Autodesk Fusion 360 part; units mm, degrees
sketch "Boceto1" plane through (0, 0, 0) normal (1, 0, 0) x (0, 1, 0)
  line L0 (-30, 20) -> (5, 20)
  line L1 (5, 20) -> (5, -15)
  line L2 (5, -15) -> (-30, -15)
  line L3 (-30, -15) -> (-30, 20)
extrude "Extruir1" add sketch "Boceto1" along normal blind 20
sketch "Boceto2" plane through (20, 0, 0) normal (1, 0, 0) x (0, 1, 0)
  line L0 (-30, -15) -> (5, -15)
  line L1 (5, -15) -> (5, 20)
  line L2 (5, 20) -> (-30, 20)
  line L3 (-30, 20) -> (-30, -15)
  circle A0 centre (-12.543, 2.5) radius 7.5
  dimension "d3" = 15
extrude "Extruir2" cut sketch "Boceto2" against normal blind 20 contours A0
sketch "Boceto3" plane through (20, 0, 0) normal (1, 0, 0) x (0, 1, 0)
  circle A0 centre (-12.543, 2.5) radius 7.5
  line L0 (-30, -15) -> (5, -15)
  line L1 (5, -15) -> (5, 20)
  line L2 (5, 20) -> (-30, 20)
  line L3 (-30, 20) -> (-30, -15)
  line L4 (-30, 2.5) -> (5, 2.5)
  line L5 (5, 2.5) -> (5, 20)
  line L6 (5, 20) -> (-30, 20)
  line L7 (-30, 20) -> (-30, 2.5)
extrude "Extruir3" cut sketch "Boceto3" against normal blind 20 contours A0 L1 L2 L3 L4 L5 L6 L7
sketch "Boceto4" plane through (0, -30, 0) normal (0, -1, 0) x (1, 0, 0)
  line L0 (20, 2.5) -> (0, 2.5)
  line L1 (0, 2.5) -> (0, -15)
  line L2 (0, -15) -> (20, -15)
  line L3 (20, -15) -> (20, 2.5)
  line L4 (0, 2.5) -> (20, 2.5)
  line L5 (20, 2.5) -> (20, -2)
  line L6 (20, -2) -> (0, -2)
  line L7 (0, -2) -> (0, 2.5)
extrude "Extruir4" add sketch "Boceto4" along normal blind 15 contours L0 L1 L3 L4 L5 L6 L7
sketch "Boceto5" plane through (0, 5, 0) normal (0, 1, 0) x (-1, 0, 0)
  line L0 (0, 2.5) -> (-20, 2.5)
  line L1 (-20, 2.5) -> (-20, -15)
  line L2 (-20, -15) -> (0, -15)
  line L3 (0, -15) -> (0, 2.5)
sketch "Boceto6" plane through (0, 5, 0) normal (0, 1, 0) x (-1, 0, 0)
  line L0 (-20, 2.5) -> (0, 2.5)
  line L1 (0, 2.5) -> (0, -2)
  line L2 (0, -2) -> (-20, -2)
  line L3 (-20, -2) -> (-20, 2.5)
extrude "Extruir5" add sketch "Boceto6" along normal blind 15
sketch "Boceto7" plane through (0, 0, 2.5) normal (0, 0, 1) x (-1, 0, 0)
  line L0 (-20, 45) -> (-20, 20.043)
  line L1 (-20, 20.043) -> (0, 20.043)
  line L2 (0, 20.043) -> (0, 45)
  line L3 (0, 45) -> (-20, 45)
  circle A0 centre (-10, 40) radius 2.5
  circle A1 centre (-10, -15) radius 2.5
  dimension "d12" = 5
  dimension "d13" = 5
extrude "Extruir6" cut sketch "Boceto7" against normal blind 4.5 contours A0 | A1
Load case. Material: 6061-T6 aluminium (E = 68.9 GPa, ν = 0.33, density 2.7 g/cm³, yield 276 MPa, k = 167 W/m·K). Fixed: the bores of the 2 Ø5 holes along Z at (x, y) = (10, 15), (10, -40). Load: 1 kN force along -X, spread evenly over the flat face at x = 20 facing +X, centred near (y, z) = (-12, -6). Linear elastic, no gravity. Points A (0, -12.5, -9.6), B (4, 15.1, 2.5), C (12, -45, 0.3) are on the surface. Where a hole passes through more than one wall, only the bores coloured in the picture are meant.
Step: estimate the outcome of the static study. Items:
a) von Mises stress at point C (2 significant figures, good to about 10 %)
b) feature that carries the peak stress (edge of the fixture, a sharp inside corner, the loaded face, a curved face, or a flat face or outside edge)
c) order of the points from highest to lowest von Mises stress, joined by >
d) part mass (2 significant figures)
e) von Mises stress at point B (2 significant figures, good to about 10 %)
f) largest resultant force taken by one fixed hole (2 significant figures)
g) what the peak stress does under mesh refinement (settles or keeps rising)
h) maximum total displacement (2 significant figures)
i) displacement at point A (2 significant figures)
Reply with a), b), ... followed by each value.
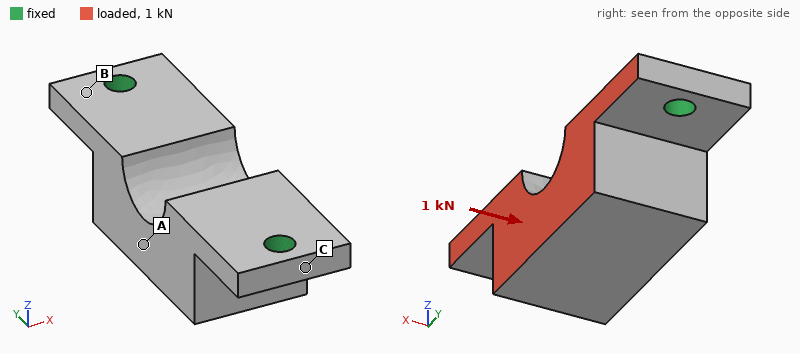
a) 16 MPa
b) edge of the fixture
c) B > C > A
d) 35 g
e) 25 MPa
f) 500 N
g) keeps rising
h) 40 µm
i) 31 µm
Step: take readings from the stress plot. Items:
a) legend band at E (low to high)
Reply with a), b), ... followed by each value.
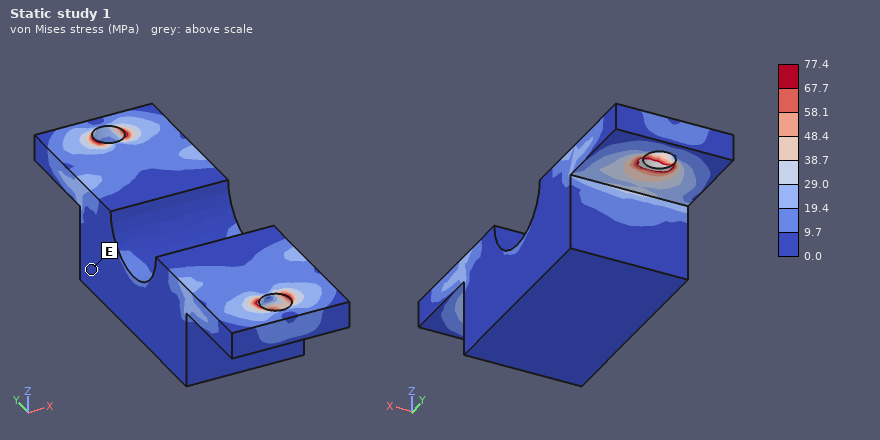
a) 0.0 to 9.7 MPa
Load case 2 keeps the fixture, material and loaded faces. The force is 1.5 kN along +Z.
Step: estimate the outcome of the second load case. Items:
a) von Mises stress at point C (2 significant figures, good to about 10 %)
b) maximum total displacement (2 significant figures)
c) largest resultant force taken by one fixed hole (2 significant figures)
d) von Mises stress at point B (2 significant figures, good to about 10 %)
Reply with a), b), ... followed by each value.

a) 47 MPa
b) 84 µm
c) 910 N
d) 34 MPa
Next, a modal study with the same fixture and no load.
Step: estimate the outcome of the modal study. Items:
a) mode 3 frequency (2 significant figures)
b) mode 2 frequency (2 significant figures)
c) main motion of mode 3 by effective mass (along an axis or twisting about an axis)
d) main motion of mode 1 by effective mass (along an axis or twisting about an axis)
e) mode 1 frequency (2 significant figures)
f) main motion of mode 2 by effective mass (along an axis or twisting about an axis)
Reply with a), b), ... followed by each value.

a) 14 kHz
b) 8800 Hz
c) along Y
d) along X
e) 4800 Hz
f) along Z
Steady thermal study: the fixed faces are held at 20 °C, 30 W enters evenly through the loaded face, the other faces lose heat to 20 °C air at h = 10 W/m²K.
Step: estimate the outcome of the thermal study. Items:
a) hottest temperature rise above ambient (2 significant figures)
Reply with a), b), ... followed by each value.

a) 15 K
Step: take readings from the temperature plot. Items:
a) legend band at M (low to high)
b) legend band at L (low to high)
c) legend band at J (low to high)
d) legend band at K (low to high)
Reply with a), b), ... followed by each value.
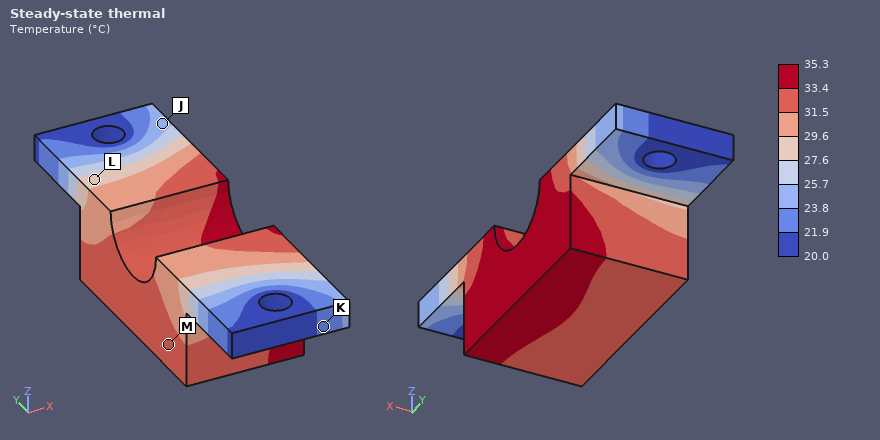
a) 31.5 to 33.4 °C
b) 27.6 to 29.6 °C
c) 23.8 to 25.7 °C
d) 21.9 to 23.8 °C
